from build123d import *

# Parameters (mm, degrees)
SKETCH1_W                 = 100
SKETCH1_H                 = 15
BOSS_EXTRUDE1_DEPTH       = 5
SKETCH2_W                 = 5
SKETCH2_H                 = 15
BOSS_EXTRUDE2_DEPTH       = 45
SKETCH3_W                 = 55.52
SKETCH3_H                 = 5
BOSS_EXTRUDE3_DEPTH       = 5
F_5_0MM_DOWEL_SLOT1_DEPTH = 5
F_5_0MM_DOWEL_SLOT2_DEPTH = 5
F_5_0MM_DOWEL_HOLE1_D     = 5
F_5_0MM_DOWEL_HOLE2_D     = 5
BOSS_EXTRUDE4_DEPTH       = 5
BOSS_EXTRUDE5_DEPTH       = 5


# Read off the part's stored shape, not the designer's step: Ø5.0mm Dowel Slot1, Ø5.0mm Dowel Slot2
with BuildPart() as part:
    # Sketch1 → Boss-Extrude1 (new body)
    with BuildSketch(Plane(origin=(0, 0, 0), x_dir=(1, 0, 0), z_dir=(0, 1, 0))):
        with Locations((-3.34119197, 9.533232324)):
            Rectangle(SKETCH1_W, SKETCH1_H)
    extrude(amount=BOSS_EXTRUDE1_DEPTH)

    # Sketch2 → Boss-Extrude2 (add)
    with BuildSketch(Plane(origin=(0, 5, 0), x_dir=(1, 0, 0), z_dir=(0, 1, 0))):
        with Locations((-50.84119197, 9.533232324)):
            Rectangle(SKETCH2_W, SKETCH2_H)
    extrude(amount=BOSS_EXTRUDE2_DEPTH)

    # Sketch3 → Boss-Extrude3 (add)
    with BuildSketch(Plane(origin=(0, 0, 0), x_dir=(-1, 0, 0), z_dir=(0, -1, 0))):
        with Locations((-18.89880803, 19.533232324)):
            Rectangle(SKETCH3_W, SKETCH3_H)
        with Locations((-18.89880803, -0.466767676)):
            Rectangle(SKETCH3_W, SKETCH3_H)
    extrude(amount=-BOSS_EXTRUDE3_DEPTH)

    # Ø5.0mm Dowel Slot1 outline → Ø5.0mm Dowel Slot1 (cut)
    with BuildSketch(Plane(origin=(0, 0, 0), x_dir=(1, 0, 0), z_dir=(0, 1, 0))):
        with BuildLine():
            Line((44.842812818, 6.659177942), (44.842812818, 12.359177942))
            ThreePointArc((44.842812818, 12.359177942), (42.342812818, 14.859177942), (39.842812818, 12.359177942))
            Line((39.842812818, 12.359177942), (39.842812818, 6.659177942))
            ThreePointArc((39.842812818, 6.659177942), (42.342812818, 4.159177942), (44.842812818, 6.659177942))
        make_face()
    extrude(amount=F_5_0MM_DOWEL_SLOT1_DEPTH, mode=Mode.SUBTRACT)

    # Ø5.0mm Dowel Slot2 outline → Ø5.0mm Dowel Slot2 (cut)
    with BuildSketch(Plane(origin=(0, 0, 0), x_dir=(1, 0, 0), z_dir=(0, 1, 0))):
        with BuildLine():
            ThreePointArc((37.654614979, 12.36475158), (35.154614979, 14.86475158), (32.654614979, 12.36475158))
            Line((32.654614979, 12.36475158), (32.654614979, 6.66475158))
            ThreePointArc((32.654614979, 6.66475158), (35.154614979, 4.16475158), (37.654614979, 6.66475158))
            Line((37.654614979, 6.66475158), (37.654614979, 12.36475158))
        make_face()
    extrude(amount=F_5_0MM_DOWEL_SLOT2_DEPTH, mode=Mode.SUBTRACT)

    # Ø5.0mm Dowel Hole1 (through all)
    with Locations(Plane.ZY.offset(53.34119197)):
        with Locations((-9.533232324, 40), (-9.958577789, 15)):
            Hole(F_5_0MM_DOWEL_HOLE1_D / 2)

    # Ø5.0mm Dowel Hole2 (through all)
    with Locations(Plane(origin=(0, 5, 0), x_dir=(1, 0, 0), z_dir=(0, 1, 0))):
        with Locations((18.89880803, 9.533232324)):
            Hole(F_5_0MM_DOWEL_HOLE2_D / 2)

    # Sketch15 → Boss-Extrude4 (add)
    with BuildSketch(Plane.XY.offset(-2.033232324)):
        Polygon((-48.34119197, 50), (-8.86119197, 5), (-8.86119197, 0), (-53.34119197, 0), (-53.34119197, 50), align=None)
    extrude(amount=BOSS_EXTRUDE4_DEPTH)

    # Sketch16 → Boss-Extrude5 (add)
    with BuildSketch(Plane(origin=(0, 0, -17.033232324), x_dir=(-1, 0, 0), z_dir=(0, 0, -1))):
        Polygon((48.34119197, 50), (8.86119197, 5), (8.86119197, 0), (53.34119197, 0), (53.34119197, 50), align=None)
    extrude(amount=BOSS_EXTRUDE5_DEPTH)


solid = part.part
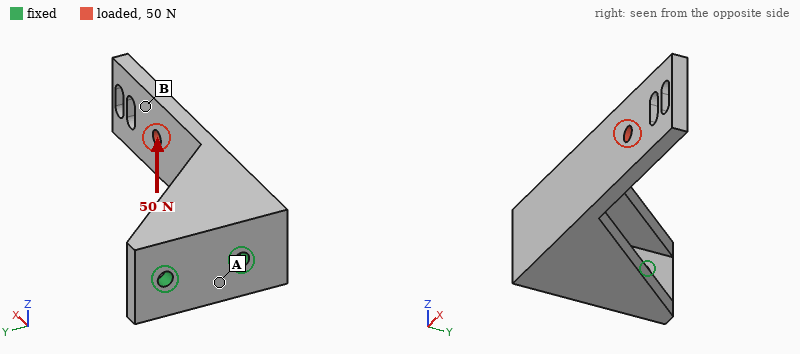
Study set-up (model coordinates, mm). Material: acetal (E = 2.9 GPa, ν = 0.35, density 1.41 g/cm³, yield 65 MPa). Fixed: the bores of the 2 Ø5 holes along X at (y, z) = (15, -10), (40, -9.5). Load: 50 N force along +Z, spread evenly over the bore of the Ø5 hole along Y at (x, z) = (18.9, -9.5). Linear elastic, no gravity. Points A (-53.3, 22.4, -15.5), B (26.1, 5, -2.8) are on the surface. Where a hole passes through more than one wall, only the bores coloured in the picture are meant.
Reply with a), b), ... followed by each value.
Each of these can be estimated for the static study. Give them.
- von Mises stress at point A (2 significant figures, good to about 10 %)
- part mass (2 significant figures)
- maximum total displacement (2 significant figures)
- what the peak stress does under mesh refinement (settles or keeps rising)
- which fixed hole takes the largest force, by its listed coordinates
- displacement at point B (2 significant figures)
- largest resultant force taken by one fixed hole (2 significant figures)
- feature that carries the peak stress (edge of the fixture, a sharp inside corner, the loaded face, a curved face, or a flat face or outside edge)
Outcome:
a) 4.8 MPa
b) 37 g
c) 1.4 mm
d) keeps rising
e) (15, -10)
f) 1.1 mm
g) 66 N
h) edge of the fixture
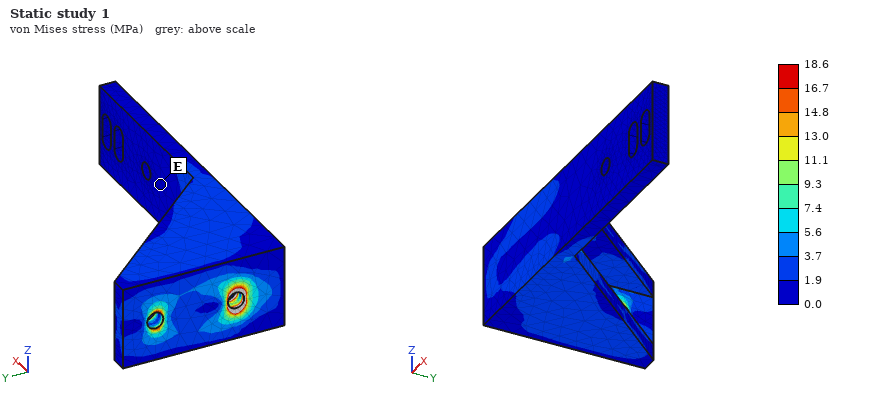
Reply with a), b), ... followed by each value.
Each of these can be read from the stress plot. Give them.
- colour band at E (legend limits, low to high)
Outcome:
a) 0.0 to 1.9 MPa
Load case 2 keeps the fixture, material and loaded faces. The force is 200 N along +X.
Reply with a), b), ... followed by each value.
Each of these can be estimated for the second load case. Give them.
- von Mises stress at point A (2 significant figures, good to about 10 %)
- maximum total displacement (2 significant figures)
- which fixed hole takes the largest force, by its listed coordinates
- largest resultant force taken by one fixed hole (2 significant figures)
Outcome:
a) 1.7 MPa
b) 0.31 mm
c) (15, -10)
d) 270 N
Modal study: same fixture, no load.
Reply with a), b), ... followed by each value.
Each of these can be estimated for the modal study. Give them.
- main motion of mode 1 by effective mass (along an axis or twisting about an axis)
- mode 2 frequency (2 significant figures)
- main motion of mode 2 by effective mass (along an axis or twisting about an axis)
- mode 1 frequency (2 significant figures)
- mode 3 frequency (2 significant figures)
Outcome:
a) along Y
b) 350 Hz
c) along Z
d) 320 Hz
e) 1300 Hz
